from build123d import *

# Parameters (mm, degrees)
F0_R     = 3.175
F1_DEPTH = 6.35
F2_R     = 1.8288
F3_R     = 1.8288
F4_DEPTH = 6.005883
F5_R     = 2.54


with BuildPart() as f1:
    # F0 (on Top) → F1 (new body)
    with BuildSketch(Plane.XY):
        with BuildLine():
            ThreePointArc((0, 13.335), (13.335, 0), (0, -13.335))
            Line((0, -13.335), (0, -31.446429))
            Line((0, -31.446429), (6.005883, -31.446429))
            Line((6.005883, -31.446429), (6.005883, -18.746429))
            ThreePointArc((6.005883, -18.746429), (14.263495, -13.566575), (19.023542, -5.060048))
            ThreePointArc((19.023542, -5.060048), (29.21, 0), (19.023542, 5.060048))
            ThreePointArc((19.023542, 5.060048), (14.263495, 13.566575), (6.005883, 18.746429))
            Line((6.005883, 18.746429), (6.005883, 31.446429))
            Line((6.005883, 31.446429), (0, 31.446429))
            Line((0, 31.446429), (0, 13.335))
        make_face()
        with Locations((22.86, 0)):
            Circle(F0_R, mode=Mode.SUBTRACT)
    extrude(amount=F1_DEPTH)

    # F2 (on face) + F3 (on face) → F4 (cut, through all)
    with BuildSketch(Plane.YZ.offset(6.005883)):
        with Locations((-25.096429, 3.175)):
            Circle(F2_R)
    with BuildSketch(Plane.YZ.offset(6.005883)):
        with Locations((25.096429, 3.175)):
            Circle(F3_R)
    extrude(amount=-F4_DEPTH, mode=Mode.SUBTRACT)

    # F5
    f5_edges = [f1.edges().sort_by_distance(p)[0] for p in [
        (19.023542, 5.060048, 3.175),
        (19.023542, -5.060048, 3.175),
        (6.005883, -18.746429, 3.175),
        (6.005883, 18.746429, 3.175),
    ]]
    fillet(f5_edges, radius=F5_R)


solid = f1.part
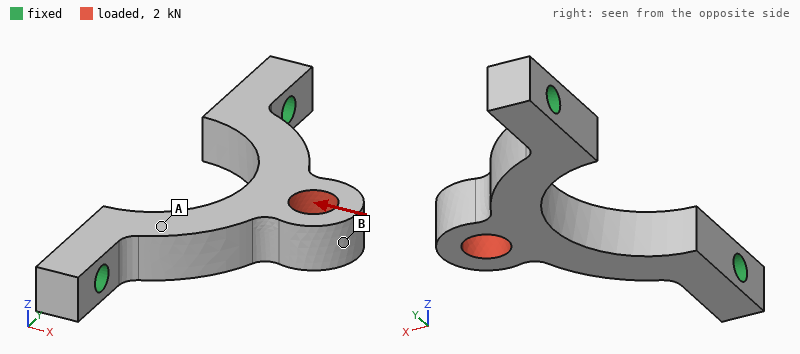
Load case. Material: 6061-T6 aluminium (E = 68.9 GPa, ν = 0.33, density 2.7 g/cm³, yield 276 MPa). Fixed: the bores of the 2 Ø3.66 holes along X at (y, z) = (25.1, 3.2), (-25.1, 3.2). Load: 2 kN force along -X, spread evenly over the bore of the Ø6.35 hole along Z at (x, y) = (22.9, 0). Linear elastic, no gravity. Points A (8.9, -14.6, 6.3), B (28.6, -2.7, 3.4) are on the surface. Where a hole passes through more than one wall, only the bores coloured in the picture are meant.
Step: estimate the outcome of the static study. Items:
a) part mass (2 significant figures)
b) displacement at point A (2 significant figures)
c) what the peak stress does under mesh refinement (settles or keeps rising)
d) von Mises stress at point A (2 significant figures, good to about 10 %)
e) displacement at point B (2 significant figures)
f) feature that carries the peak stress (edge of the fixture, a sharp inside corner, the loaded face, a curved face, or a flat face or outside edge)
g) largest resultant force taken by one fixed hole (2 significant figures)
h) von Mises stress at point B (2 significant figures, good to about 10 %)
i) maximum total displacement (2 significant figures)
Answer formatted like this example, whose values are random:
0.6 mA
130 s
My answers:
9.1 g
16 µm
keeps rising
43 MPa
32 µm
edge of the fixture
1.4 kN
16 MPa
33 µm
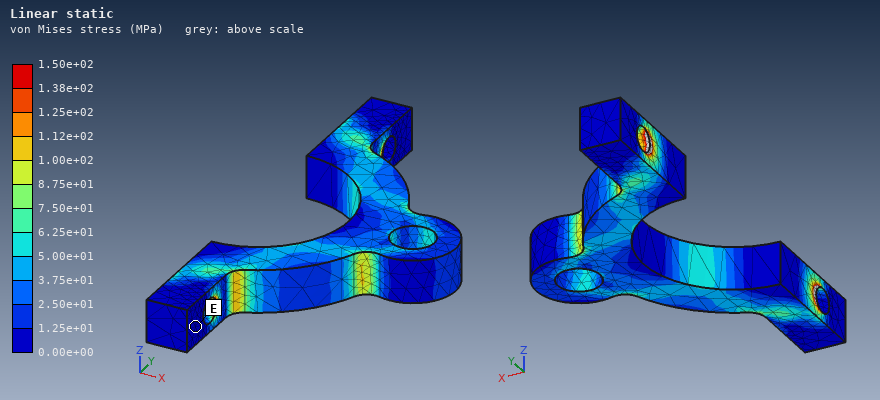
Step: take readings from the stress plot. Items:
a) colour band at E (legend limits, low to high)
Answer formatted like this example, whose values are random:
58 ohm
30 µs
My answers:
0.00e+00 to 1.25e+01 MPa
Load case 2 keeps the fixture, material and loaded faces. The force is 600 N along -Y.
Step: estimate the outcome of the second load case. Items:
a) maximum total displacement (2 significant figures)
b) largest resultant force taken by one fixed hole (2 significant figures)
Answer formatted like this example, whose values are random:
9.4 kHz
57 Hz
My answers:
17 µm
420 N
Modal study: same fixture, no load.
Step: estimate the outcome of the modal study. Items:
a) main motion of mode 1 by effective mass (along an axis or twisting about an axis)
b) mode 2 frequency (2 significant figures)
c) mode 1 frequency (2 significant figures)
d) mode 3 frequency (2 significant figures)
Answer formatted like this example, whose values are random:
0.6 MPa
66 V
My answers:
along Z
18 kHz
4500 Hz
18 kHz
